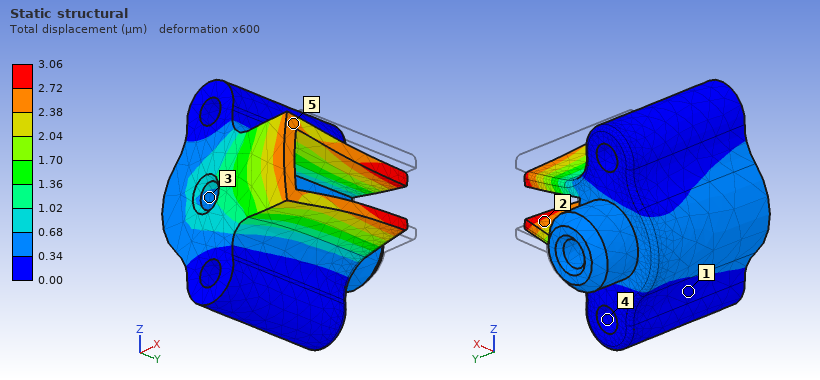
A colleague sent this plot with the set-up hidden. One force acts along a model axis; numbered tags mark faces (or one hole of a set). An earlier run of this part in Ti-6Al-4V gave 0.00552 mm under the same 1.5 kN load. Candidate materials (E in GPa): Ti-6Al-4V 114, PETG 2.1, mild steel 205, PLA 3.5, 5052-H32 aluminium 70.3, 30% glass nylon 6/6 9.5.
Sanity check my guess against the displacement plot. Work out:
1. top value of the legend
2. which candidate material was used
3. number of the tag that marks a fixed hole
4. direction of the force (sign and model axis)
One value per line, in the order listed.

3.06 µm
mild steel
4
-X
